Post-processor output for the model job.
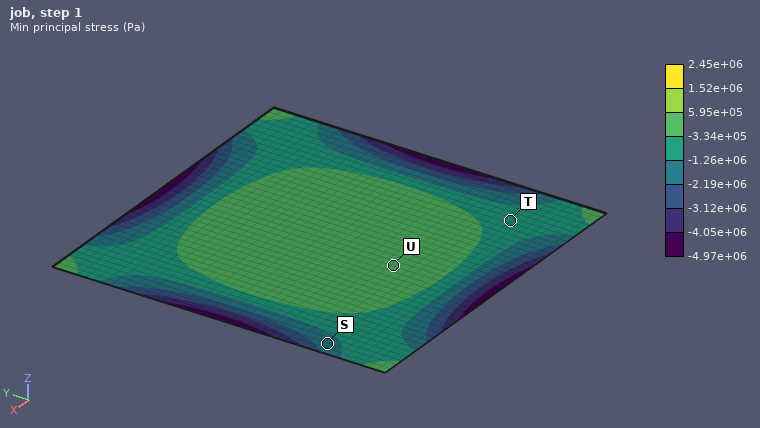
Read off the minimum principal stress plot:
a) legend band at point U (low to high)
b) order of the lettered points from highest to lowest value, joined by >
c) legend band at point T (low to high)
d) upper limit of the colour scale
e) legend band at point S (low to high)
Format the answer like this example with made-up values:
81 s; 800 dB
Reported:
-3.34e+05 to 5.95e+05 Pa; U > T > S; -1.26e+06 to -3.34e+05 Pa; 2.45e+06 Pa; -2.19e+06 to -1.26e+06 Pa
